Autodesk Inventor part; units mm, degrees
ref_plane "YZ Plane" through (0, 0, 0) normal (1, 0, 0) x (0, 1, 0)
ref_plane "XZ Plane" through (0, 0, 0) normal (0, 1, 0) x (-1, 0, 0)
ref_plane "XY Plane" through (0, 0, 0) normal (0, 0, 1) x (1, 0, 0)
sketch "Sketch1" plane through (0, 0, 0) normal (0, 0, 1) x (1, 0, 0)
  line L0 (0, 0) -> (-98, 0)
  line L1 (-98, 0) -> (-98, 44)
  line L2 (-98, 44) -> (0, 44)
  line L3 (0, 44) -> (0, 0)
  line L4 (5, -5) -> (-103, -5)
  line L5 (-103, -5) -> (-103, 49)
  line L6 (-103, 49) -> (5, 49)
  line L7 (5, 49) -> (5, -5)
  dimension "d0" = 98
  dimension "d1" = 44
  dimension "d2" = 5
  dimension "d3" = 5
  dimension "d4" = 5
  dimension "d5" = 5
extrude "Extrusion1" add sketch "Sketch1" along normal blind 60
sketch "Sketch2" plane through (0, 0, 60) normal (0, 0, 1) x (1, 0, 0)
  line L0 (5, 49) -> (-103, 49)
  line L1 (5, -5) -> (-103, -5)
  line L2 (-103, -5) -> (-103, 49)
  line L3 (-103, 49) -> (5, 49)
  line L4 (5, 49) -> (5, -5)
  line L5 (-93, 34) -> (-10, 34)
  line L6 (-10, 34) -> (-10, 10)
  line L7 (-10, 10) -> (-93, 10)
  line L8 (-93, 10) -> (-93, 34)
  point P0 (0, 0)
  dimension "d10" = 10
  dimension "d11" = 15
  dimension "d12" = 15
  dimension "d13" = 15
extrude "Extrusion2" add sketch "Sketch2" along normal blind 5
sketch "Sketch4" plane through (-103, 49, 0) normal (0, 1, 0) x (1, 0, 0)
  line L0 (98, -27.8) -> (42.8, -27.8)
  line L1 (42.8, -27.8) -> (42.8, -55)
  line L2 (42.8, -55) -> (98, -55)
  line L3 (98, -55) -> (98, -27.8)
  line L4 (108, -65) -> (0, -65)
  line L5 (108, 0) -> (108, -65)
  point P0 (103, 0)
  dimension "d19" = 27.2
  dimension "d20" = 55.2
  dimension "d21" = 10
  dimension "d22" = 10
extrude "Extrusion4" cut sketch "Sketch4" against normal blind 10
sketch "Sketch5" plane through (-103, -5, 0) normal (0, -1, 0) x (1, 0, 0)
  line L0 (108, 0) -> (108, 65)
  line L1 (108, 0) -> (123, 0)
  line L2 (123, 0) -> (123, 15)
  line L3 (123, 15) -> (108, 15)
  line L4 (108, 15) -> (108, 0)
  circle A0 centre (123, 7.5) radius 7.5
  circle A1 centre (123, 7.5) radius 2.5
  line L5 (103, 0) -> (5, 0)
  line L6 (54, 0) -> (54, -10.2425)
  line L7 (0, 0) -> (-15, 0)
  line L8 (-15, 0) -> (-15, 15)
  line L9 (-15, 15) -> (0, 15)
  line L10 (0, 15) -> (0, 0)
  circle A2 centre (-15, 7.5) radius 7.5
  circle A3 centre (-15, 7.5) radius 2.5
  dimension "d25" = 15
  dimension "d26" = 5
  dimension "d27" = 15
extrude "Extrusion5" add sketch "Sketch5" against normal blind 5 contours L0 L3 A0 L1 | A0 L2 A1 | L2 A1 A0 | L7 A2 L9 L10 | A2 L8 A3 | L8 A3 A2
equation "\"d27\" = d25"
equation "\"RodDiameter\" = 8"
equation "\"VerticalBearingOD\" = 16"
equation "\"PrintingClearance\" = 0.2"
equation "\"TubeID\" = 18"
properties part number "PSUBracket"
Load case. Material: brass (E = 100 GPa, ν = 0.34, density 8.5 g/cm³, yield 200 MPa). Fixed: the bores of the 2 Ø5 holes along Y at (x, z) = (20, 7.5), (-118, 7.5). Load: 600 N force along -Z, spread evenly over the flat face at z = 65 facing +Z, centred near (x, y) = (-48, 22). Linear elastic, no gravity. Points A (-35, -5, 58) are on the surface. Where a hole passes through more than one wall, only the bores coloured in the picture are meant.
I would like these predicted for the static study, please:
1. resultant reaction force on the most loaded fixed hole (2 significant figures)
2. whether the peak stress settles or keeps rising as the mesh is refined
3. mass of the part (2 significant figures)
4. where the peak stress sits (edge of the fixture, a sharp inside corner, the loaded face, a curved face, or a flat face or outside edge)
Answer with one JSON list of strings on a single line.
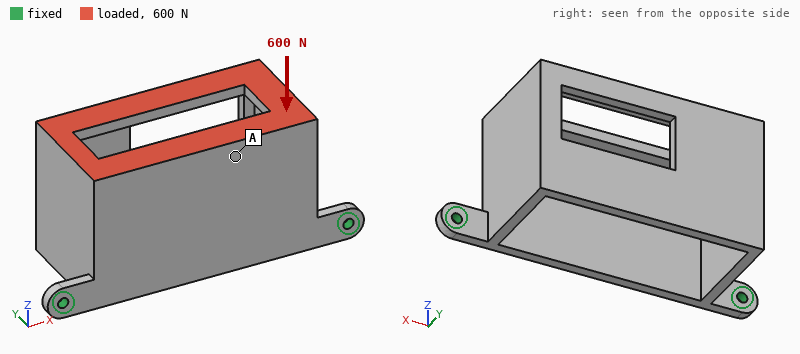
["320 N", "keeps rising", "900 g", "edge of the fixture"]
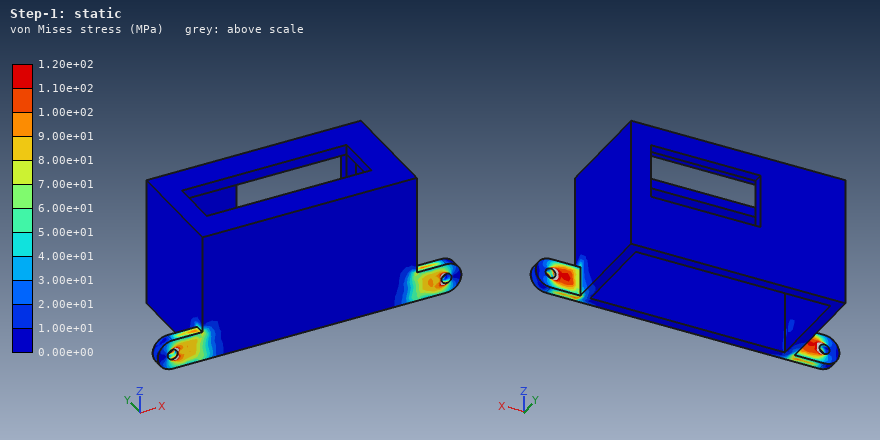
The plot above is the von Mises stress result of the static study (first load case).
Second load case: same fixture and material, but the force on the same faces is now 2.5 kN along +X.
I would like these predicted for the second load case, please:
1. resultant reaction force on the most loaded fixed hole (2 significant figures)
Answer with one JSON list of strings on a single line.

["1.8 kN"]
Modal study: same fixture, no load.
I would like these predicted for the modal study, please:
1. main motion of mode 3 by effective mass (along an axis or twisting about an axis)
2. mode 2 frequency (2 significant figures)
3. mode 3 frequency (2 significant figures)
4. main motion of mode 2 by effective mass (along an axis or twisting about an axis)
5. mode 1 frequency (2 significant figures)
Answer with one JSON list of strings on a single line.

["along Y", "600 Hz", "1100 Hz", "along X", "190 Hz"]
